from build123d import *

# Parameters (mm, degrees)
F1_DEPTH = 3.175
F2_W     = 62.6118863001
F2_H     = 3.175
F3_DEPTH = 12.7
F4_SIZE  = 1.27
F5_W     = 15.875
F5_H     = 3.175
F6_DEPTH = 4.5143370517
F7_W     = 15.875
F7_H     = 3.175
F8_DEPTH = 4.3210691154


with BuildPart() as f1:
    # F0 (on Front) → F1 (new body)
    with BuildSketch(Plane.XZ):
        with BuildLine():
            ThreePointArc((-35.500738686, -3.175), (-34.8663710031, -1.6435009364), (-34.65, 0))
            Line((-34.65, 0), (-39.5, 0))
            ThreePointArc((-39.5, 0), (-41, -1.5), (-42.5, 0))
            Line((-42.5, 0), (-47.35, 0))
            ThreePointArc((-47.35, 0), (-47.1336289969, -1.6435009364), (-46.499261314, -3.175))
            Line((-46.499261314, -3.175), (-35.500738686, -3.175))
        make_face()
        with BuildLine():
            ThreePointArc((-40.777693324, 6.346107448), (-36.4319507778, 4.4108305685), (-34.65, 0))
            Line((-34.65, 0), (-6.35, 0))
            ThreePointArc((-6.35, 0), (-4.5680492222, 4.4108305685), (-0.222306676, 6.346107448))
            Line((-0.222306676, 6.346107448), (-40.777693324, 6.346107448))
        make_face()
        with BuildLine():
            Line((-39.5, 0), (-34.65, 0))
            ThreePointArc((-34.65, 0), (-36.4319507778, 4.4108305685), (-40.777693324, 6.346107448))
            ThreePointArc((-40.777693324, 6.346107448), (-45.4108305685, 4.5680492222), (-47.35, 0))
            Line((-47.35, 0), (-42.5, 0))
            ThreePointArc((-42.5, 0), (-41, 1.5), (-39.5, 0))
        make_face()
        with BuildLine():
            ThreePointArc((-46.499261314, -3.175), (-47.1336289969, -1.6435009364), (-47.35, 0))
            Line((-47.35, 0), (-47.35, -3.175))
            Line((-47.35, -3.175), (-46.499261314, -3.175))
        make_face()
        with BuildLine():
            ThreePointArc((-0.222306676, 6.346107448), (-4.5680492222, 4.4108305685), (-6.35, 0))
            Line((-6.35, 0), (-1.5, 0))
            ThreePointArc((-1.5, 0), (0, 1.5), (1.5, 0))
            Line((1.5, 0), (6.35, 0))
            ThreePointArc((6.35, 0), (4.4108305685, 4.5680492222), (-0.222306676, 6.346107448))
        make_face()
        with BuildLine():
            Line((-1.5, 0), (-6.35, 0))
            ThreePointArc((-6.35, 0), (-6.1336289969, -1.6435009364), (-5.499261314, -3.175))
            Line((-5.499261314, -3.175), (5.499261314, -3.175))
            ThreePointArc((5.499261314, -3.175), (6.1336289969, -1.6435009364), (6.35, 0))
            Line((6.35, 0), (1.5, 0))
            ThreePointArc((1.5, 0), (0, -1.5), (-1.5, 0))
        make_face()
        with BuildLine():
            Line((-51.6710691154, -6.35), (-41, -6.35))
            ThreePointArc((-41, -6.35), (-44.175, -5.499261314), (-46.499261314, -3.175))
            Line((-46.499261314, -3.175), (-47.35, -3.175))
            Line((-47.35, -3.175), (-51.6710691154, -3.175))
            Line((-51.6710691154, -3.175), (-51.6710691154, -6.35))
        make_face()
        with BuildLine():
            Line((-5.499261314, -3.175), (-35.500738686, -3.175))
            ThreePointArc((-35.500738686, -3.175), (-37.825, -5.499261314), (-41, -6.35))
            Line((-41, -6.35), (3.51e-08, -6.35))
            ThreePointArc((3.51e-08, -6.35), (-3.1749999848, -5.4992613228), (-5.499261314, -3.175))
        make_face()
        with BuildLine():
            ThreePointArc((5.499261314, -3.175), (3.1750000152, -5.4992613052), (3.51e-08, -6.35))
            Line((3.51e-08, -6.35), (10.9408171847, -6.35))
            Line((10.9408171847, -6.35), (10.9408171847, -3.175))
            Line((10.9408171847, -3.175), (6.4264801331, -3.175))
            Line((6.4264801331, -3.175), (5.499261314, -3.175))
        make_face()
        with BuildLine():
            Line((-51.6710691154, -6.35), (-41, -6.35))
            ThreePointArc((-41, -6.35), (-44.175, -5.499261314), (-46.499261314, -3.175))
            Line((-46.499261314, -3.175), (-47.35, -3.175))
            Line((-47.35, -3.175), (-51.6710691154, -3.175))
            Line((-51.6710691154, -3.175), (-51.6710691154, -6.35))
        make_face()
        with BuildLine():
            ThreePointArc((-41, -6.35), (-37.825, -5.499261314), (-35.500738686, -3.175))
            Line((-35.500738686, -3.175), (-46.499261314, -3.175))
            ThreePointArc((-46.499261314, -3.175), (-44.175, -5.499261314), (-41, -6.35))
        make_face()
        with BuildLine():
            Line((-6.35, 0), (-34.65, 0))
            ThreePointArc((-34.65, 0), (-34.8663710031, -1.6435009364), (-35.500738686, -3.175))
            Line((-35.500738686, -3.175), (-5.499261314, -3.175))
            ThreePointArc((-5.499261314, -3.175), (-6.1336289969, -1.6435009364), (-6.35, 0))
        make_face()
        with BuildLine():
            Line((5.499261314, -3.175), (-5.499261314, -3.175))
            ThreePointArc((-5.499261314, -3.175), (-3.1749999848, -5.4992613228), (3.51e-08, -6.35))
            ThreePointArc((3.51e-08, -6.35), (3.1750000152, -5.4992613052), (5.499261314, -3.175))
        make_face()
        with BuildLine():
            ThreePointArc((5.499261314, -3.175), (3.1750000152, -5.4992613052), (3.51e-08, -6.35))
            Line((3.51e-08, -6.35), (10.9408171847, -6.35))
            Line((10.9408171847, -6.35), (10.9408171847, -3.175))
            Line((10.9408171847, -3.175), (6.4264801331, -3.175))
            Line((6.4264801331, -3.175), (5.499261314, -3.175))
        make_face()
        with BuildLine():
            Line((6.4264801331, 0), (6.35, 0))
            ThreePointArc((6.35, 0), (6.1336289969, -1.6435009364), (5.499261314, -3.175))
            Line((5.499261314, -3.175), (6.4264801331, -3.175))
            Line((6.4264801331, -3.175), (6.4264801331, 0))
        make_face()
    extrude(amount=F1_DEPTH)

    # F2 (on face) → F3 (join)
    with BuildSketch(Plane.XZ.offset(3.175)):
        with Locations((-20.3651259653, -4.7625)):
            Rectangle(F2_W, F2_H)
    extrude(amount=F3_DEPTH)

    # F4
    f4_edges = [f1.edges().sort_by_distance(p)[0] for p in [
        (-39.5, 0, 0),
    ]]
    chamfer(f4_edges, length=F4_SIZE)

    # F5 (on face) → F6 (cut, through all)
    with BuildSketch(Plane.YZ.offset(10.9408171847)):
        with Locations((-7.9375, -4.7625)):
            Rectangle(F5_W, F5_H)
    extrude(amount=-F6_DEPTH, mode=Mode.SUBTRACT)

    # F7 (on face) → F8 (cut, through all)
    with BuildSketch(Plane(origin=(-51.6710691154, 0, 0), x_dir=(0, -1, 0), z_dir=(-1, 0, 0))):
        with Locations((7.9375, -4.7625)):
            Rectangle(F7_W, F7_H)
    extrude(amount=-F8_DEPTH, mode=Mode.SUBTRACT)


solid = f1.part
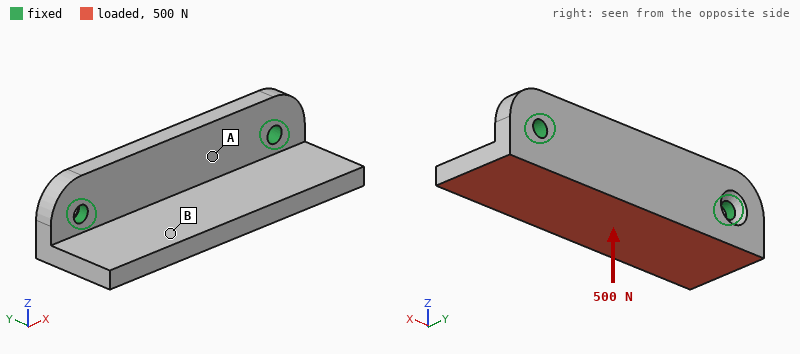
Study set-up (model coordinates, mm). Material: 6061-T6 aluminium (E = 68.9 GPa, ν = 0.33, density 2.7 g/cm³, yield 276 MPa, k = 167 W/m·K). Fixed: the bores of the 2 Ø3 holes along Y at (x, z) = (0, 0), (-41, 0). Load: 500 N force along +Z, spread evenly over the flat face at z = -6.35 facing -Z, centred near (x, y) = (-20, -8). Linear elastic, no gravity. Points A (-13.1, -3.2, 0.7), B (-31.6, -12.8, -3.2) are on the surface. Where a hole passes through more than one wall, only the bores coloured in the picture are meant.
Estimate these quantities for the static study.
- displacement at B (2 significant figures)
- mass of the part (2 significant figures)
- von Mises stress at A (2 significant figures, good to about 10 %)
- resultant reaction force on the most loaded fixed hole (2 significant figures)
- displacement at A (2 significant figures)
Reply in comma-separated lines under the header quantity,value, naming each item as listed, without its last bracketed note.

quantity,value
displacement at B,49 µm
mass of the part,11 g
von Mises stress at A,21 MPa
resultant reaction force on the most loaded fixed hole,250 N
displacement at A,10 µm
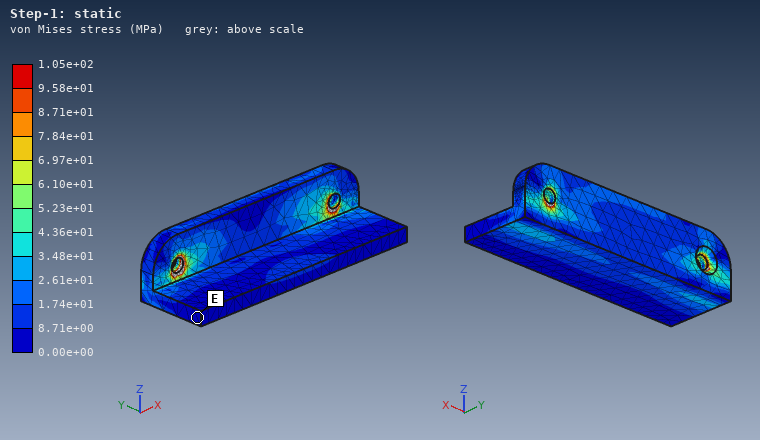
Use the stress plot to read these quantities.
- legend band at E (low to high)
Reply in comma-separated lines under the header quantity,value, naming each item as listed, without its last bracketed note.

quantity,value
legend band at E,0.00e+00 to 8.71e+00 MPa
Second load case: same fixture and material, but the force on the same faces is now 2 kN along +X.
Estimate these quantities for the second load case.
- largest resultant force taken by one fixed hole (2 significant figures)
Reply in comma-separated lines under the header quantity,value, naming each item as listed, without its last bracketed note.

quantity,value
largest resultant force taken by one fixed hole,1.1 kN
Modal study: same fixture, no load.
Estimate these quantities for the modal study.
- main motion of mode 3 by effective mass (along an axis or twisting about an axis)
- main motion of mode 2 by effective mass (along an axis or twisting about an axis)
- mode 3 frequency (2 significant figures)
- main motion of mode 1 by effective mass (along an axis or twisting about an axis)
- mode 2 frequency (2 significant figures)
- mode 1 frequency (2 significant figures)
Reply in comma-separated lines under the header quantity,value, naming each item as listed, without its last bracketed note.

quantity,value
main motion of mode 3 by effective mass,along Y
main motion of mode 2 by effective mass,twisting about Y
mode 3 frequency,14 kHz
main motion of mode 1 by effective mass,along Z
mode 2 frequency,10 kHz
mode 1 frequency,6100 Hz
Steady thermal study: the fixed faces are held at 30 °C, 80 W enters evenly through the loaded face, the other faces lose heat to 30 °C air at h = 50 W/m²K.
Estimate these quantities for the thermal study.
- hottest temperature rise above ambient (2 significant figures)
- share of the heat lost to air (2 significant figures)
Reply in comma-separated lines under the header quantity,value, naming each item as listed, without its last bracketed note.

quantity,value
hottest temperature rise above ambient,52 K
share of the heat lost to air,4.4 %
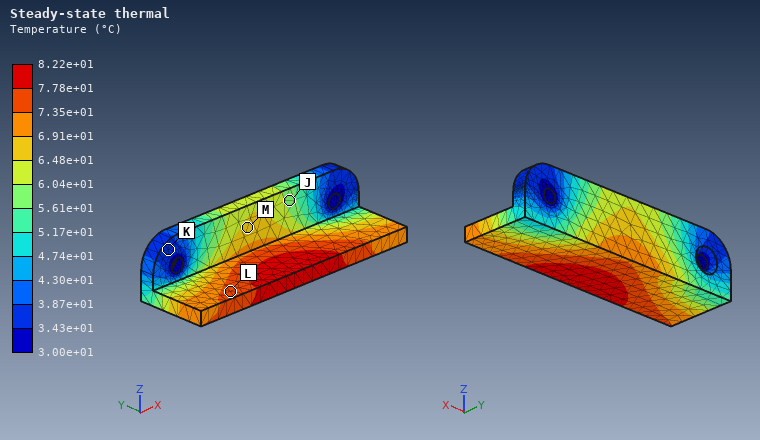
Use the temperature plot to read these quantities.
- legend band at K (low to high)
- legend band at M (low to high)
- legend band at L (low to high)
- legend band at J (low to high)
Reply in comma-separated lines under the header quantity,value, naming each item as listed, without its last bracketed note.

quantity,value
legend band at K,3.43e+01 to 3.87e+01 °C
legend band at M,6.48e+01 to 6.91e+01 °C
legend band at L,7.35e+01 to 7.78e+01 °C
legend band at J,5.61e+01 to 6.04e+01 °C
